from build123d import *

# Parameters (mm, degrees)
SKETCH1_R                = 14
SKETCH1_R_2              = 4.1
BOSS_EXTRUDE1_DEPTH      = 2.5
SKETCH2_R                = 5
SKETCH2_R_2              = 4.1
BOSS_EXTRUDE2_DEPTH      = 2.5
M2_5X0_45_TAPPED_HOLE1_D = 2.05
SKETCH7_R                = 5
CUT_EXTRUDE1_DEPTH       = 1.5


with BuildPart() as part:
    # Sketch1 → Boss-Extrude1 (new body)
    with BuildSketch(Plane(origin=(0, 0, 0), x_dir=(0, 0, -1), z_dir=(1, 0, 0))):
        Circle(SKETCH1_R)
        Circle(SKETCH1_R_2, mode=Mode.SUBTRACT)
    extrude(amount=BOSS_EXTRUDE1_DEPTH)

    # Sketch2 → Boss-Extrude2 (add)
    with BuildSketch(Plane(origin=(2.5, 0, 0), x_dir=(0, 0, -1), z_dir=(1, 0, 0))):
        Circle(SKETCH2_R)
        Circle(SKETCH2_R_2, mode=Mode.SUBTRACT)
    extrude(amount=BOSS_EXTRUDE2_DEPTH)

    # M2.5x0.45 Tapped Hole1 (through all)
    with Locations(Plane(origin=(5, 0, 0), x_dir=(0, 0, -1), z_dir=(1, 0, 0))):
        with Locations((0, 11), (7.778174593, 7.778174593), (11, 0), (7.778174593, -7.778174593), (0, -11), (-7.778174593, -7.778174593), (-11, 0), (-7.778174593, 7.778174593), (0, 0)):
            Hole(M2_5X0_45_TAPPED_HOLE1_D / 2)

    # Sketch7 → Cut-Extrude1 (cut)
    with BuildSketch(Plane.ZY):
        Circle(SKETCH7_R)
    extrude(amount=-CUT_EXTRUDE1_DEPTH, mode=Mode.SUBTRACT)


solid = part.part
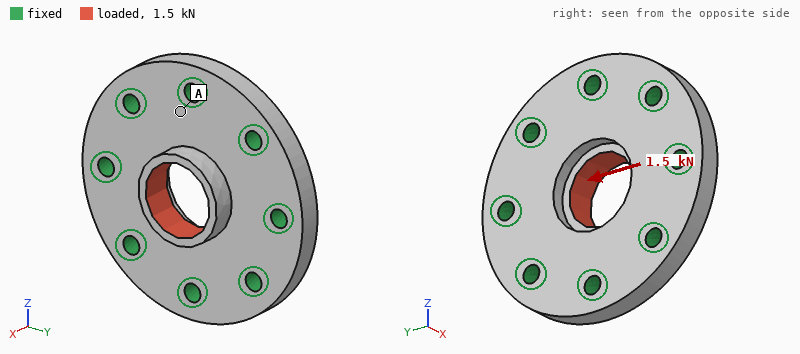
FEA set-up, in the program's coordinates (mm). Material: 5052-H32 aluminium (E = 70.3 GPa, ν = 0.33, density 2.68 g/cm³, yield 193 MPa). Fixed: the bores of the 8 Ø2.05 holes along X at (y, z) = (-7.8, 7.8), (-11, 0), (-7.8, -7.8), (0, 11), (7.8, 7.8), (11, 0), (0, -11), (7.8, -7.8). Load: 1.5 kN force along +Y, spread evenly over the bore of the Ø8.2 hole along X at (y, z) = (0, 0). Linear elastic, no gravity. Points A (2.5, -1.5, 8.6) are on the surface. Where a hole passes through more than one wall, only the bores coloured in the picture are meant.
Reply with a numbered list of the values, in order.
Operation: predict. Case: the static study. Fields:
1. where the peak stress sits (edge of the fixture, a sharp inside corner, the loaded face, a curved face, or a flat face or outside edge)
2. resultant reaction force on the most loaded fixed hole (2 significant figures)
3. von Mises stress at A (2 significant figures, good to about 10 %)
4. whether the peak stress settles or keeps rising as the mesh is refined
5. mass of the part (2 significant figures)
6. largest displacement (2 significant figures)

1. a sharp inside corner
2. 310 N
3. 13 MPa
4. keeps rising
5. 3.7 g
6. 14 µm
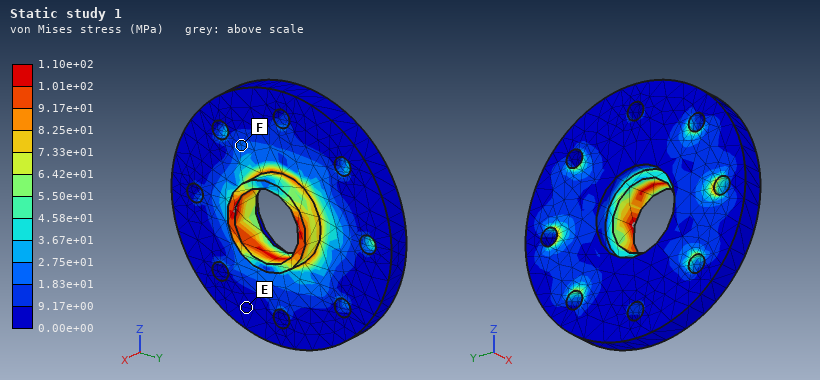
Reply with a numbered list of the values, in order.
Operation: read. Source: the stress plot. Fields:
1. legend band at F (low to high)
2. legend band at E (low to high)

1. 1.83e+01 to 2.75e+01 MPa
2. 0.00e+00 to 9.17e+00 MPa
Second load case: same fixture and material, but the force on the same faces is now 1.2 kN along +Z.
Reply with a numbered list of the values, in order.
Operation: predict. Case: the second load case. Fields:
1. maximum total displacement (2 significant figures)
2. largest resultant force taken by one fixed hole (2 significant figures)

1. 11 µm
2. 250 N
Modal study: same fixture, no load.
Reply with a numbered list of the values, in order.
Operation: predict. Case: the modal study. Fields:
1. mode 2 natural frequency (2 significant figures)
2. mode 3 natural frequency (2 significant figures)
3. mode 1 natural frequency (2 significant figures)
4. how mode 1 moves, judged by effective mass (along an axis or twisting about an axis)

1. 74 kHz
2. 74 kHz
3. 57 kHz
4. along X
